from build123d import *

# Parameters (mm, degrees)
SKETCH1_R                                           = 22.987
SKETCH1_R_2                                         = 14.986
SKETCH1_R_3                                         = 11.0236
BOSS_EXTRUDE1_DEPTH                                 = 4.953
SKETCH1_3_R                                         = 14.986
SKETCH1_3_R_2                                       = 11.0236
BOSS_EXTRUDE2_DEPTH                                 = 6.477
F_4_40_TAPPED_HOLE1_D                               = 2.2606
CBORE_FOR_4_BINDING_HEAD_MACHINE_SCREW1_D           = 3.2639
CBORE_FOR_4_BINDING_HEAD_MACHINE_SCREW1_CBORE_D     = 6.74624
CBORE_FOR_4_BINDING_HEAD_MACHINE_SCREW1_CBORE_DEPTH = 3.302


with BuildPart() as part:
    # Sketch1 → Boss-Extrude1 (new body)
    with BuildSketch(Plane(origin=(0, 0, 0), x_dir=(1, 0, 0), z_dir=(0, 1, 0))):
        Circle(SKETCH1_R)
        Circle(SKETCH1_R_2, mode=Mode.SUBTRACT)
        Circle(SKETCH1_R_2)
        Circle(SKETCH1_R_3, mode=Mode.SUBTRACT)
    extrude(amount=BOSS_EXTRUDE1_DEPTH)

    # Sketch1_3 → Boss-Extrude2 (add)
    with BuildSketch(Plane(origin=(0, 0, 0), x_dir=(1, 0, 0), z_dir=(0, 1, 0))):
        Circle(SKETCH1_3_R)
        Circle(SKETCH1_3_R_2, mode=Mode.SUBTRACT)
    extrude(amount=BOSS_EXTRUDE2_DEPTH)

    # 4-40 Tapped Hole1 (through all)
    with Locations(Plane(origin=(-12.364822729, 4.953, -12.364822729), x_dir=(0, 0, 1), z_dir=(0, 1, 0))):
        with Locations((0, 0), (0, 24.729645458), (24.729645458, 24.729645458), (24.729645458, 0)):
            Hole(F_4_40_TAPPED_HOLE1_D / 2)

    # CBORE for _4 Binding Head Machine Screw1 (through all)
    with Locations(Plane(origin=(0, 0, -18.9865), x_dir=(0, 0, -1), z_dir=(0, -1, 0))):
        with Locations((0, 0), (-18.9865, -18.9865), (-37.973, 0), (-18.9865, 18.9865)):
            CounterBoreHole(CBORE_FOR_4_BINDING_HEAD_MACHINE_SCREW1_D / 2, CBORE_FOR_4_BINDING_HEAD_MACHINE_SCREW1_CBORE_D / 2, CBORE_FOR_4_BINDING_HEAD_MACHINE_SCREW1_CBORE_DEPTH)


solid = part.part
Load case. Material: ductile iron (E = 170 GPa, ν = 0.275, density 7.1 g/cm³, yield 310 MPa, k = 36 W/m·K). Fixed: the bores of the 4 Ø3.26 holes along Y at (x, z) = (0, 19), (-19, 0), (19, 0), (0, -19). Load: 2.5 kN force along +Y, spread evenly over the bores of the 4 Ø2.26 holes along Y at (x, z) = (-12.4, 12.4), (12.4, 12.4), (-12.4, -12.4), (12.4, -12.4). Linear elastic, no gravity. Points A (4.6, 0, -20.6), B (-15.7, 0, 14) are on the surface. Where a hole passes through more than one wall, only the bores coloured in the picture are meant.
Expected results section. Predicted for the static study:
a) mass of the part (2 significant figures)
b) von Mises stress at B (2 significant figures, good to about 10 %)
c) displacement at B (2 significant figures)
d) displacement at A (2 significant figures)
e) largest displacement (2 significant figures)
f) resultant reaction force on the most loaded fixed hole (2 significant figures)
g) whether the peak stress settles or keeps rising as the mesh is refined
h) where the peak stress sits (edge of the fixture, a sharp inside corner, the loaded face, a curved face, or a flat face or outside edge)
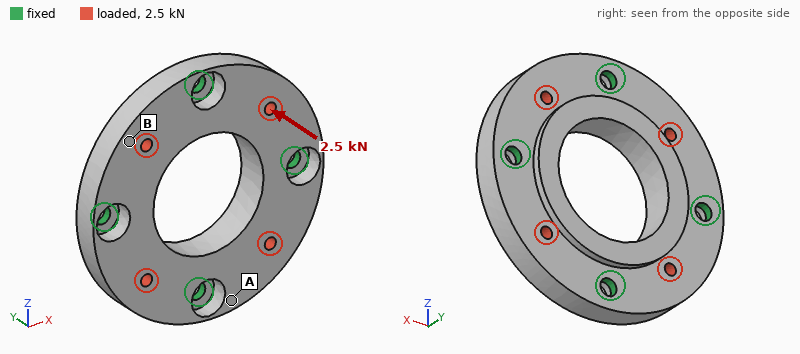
44 g
43 MPa
7.6 µm
2.6 µm
8.3 µm
660 N
keeps rising
edge of the fixture
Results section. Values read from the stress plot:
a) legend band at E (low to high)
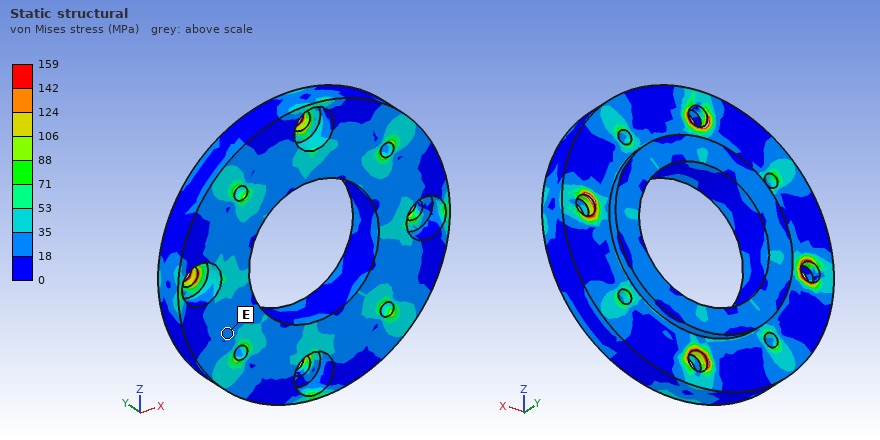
18 to 35 MPa
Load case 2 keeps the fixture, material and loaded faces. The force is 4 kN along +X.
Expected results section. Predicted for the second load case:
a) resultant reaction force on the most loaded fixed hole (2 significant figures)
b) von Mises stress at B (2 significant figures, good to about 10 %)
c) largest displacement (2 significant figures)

1.2 kN
16 MPa
4.3 µm
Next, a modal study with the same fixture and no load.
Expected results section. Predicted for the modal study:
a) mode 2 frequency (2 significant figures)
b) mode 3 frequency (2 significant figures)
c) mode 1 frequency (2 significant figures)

17 kHz
17 kHz
14 kHz
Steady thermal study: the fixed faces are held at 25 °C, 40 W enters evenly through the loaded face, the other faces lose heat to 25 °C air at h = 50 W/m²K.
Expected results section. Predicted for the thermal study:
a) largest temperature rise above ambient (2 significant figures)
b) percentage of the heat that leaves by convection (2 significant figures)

54 K
16 %
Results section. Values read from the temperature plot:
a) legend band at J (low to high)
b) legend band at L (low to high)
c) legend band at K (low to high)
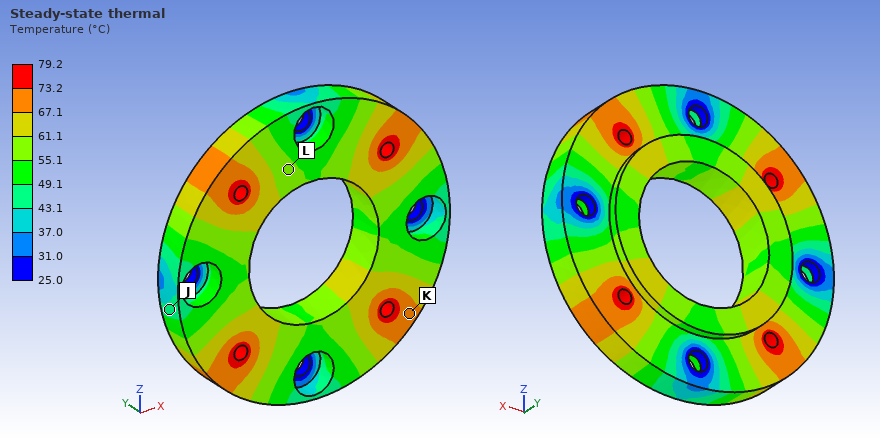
43.1 to 49.1 °C
55.1 to 61.1 °C
67.1 to 73.2 °C
